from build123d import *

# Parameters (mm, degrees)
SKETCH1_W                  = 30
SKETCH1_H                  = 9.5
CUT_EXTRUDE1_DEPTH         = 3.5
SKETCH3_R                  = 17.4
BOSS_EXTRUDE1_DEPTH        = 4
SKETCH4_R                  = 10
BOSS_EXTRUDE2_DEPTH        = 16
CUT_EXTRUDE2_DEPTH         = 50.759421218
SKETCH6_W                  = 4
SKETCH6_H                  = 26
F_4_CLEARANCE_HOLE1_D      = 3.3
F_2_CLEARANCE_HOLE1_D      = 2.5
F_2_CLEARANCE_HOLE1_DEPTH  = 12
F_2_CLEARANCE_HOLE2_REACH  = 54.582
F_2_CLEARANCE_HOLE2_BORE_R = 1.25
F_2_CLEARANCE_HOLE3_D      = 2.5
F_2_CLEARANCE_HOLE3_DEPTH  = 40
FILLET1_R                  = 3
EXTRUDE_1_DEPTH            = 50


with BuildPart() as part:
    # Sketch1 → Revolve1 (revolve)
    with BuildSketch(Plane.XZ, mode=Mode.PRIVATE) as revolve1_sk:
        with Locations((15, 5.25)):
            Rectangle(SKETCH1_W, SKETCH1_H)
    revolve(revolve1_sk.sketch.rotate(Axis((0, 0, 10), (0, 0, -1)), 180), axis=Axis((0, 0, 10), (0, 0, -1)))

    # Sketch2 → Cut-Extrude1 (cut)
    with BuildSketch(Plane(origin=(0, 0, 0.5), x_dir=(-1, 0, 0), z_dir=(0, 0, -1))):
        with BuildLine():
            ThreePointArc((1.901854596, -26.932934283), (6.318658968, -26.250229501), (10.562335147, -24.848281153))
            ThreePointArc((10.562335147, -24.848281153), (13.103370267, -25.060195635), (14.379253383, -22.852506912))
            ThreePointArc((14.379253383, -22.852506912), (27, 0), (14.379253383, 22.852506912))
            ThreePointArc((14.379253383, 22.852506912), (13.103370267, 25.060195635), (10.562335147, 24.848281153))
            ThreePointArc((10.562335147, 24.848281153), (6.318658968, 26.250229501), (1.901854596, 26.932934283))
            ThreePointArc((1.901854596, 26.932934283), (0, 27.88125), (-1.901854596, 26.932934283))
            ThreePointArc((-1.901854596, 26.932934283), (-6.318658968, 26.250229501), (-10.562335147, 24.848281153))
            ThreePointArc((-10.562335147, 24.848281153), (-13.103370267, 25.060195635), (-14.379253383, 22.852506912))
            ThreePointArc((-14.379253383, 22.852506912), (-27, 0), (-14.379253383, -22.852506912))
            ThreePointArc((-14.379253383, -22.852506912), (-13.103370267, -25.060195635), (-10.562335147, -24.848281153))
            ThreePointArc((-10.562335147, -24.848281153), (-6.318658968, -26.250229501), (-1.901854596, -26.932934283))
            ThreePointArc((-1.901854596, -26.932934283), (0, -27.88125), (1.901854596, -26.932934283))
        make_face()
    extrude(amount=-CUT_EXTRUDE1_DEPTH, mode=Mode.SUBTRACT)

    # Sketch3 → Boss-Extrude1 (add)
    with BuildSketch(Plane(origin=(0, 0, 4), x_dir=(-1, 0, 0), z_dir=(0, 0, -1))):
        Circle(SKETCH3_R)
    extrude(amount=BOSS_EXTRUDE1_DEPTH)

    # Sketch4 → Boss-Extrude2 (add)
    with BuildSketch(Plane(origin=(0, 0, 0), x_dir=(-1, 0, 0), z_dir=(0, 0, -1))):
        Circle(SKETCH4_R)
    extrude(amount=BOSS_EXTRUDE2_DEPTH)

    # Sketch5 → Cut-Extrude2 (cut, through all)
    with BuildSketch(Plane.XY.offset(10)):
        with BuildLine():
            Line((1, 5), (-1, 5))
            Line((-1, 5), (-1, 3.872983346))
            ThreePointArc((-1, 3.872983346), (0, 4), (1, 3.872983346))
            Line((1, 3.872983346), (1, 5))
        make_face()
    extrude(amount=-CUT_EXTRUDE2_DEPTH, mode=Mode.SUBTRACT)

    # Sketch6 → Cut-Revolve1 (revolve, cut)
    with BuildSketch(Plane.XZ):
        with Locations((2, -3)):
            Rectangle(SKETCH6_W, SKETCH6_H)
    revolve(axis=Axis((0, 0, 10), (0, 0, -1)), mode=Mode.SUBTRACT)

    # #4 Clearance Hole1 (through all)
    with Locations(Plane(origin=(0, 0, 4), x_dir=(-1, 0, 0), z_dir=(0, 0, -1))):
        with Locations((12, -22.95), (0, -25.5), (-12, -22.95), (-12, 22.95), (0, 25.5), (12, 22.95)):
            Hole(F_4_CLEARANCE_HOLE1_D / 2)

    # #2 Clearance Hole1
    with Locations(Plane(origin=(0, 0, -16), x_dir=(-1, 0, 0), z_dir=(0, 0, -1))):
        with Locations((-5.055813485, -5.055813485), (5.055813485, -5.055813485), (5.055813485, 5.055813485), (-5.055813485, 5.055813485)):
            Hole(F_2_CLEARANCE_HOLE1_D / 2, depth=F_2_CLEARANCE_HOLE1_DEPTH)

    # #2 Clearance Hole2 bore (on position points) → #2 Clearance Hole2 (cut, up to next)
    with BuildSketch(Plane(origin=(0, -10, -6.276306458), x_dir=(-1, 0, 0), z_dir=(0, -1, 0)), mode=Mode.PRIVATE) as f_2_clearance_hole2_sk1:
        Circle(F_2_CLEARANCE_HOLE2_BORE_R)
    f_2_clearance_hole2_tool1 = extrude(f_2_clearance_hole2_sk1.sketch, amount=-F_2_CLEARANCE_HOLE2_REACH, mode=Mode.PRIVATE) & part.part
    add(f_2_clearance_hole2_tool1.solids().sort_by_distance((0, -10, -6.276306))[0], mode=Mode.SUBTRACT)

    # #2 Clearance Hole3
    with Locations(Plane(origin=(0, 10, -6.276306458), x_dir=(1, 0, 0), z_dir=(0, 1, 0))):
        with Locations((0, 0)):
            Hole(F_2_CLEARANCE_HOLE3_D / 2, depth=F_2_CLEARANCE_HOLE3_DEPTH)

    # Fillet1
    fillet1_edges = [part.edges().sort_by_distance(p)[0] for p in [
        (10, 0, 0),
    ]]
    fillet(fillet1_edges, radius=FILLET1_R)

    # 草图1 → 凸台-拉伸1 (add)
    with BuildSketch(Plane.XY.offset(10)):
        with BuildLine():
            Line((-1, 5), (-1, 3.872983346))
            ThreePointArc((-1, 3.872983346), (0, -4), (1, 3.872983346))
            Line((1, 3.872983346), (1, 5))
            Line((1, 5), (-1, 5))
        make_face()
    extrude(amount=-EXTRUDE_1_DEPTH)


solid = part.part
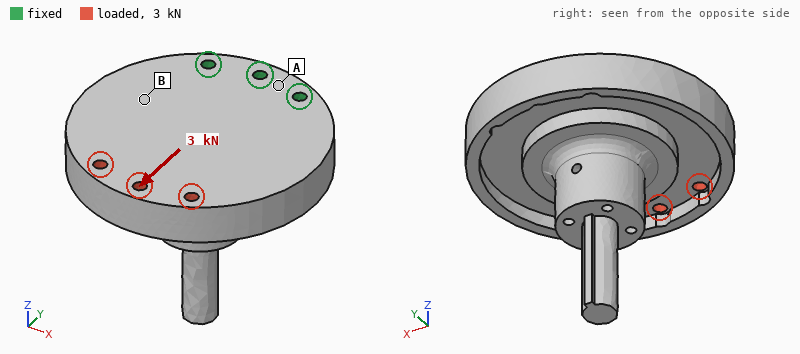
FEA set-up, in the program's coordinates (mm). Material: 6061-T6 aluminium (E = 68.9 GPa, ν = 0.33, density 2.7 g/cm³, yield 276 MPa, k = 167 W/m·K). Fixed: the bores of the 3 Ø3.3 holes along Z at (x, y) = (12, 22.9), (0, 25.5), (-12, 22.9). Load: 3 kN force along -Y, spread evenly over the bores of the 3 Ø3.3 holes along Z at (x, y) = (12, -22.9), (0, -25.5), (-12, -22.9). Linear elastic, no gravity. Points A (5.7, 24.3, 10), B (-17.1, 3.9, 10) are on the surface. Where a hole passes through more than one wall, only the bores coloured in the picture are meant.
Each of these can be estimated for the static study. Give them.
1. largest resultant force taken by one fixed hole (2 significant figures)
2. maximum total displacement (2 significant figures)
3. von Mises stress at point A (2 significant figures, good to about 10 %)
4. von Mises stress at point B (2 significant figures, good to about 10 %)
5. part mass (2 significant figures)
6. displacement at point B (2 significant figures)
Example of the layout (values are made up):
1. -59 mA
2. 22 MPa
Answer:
1. 1.1 kN
2. 22 µm
3. 4.8 MPa
4. 11 MPa
5. 77 g
6. 4.7 µm
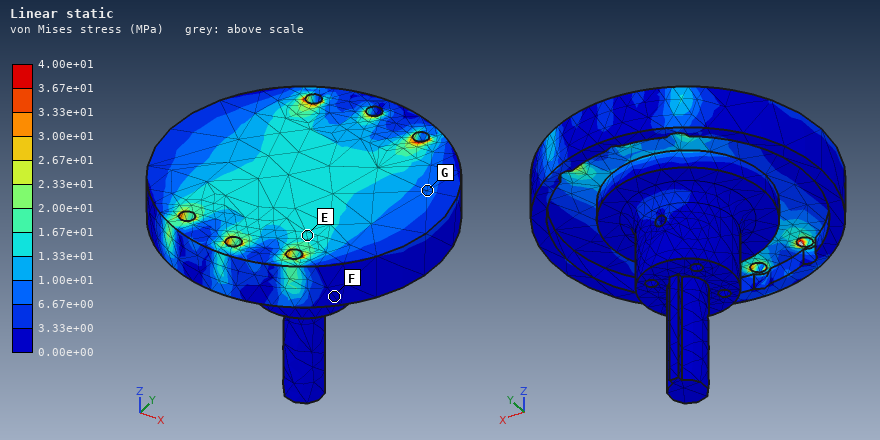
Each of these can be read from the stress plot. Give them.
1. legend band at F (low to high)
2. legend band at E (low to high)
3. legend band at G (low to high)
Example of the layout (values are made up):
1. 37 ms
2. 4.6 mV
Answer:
1. 0.00e+00 to 3.33e+00 MPa
2. 1.33e+01 to 1.67e+01 MPa
3. 6.67e+00 to 1.00e+01 MPa
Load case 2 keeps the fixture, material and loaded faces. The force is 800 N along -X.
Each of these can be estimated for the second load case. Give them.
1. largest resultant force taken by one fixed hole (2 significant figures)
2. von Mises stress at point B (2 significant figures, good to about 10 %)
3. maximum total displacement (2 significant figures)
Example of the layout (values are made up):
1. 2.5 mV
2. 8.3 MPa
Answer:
1. 1.5 kN
2. 6.3 MPa
3. 23 µm
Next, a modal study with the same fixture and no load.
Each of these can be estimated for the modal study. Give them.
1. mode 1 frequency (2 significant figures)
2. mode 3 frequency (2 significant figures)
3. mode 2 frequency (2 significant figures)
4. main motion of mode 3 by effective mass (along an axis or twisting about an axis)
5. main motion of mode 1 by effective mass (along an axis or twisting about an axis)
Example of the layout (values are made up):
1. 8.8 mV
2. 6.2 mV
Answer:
1. 1600 Hz
2. 6200 Hz
3. 4500 Hz
4. along X
5. along Z
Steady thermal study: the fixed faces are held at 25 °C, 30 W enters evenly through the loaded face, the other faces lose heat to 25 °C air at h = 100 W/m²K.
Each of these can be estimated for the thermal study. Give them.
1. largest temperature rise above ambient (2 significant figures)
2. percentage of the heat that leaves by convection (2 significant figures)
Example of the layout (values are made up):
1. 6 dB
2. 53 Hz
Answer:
1. 22 K
2. 30 %
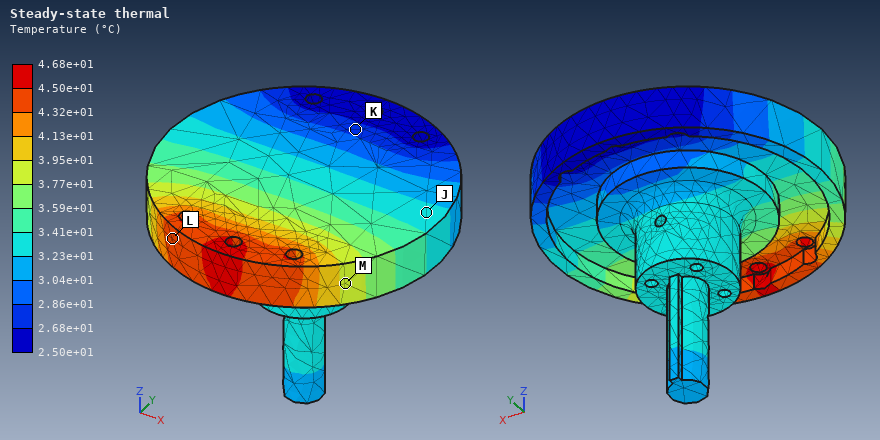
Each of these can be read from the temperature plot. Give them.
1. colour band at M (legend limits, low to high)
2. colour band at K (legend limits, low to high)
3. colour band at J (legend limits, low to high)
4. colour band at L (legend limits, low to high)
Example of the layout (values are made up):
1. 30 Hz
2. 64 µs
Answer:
1. 3.77e+01 to 3.95e+01 °C
2. 2.68e+01 to 2.86e+01 °C
3. 3.23e+01 to 3.41e+01 °C
4. 4.32e+01 to 4.50e+01 °C
